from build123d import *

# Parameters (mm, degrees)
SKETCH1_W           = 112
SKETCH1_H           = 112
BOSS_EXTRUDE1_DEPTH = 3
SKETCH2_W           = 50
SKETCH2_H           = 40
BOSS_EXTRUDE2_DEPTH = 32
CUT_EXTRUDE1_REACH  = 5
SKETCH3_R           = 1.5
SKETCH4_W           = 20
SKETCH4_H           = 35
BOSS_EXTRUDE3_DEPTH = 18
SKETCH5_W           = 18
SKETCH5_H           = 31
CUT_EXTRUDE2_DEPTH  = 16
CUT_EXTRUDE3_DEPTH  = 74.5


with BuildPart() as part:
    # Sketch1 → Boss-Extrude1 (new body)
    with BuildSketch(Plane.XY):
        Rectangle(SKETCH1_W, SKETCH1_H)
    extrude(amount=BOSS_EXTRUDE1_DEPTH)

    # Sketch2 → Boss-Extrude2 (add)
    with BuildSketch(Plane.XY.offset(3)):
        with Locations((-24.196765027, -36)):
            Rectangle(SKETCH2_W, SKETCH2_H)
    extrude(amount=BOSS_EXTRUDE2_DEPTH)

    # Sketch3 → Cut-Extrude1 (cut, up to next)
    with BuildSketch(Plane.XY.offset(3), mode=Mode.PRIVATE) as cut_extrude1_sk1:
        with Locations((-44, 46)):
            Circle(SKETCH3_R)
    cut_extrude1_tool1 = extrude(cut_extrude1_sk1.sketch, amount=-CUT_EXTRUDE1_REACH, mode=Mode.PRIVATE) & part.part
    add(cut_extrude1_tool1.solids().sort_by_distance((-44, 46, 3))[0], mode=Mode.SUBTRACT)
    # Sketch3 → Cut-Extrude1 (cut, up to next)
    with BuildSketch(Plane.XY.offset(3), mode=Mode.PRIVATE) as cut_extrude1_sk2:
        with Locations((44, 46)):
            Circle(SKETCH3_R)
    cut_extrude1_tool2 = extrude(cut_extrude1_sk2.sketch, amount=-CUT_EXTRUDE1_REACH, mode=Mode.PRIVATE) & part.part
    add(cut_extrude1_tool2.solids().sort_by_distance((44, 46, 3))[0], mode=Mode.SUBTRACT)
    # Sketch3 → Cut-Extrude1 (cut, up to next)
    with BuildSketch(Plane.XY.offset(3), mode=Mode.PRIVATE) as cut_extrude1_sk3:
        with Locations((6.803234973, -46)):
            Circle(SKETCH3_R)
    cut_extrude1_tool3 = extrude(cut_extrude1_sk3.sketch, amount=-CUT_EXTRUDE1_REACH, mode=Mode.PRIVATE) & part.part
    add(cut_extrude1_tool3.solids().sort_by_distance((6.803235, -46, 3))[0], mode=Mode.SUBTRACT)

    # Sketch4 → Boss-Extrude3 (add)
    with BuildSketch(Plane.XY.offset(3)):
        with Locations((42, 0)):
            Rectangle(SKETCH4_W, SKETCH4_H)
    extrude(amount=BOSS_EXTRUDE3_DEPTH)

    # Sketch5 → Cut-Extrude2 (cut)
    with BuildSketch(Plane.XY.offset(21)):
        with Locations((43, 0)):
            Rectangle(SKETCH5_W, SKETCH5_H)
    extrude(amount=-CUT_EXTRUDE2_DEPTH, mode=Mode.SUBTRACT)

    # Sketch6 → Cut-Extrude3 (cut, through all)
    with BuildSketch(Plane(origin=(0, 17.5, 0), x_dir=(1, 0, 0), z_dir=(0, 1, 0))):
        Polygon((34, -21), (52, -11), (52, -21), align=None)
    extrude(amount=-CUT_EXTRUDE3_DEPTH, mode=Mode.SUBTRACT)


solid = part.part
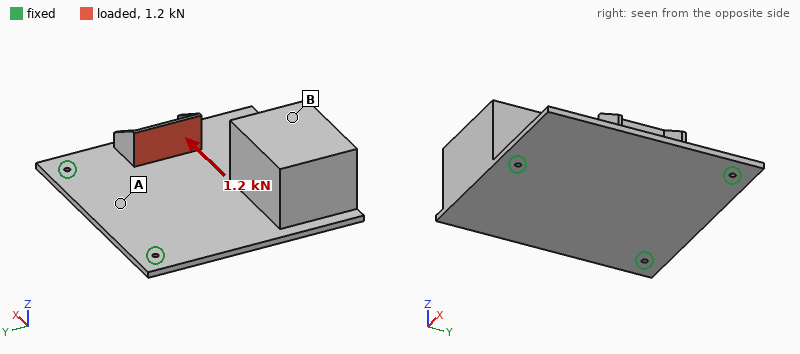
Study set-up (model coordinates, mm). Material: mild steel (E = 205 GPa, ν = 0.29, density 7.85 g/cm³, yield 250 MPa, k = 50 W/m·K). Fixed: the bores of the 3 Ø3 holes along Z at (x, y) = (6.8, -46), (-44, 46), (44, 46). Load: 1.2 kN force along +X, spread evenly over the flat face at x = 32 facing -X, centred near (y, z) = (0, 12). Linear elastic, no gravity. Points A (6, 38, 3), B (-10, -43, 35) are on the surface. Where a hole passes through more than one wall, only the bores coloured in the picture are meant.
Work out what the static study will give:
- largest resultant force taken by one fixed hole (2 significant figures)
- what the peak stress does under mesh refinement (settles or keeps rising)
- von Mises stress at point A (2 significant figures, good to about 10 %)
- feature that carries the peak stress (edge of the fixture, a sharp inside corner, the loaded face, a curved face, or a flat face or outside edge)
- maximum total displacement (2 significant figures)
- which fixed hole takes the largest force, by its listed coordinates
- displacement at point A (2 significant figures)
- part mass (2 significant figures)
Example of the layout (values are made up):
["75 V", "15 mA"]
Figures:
["490 N", "keeps rising", "19 MPa", "edge of the fixture", "0.18 mm", "(6.8, -46)", "0.032 mm", "820 g"]
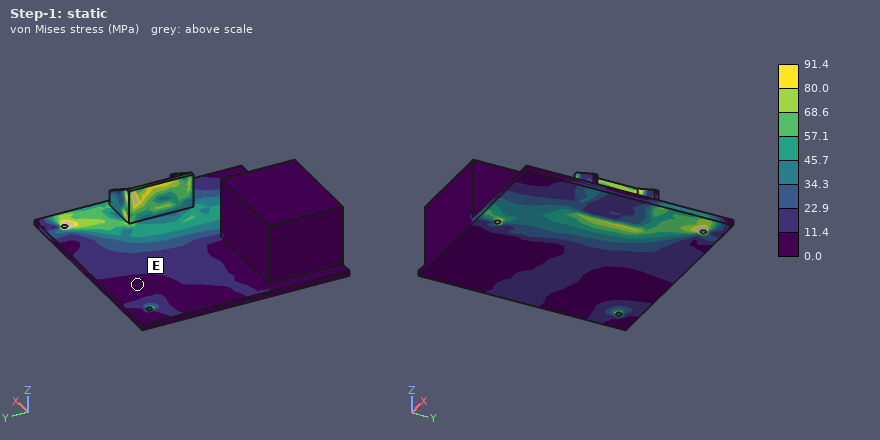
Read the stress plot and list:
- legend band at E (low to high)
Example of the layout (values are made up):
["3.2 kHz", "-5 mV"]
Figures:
["0.0 to 11.4 MPa"]
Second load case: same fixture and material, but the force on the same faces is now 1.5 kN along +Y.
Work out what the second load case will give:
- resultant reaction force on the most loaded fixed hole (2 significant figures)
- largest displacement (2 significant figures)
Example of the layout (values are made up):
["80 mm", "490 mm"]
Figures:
["740 N", "0.14 mm"]
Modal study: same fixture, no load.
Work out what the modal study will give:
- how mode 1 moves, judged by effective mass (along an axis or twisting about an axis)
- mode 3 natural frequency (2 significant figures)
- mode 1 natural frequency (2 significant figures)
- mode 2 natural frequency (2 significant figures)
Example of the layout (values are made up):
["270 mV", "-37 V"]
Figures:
["along Z", "1100 Hz", "360 Hz", "780 Hz"]
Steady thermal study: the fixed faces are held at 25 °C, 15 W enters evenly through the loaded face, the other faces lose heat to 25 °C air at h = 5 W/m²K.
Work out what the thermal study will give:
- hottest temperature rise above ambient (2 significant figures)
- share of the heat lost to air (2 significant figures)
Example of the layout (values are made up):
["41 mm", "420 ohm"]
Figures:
["71 K", "20 %"]
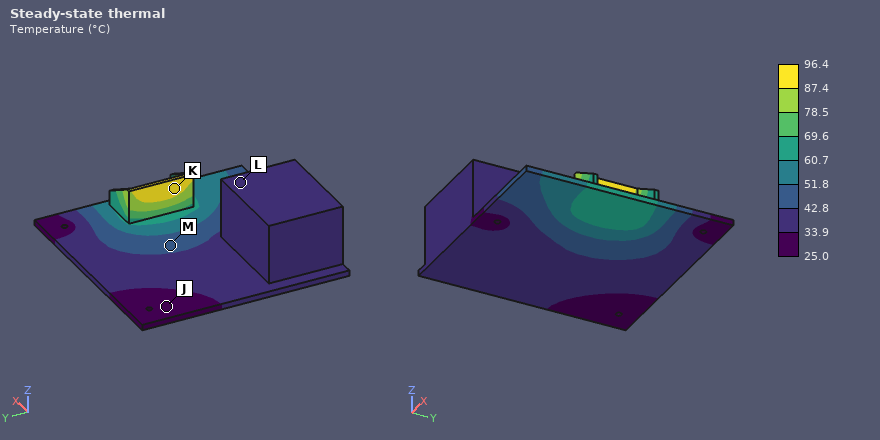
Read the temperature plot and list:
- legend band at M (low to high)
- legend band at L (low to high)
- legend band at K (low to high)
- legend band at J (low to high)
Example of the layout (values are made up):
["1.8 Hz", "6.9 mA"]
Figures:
["42.8 to 51.8 °C", "33.9 to 42.8 °C", "87.4 to 96.4 °C", "25.0 to 33.9 °C"]
